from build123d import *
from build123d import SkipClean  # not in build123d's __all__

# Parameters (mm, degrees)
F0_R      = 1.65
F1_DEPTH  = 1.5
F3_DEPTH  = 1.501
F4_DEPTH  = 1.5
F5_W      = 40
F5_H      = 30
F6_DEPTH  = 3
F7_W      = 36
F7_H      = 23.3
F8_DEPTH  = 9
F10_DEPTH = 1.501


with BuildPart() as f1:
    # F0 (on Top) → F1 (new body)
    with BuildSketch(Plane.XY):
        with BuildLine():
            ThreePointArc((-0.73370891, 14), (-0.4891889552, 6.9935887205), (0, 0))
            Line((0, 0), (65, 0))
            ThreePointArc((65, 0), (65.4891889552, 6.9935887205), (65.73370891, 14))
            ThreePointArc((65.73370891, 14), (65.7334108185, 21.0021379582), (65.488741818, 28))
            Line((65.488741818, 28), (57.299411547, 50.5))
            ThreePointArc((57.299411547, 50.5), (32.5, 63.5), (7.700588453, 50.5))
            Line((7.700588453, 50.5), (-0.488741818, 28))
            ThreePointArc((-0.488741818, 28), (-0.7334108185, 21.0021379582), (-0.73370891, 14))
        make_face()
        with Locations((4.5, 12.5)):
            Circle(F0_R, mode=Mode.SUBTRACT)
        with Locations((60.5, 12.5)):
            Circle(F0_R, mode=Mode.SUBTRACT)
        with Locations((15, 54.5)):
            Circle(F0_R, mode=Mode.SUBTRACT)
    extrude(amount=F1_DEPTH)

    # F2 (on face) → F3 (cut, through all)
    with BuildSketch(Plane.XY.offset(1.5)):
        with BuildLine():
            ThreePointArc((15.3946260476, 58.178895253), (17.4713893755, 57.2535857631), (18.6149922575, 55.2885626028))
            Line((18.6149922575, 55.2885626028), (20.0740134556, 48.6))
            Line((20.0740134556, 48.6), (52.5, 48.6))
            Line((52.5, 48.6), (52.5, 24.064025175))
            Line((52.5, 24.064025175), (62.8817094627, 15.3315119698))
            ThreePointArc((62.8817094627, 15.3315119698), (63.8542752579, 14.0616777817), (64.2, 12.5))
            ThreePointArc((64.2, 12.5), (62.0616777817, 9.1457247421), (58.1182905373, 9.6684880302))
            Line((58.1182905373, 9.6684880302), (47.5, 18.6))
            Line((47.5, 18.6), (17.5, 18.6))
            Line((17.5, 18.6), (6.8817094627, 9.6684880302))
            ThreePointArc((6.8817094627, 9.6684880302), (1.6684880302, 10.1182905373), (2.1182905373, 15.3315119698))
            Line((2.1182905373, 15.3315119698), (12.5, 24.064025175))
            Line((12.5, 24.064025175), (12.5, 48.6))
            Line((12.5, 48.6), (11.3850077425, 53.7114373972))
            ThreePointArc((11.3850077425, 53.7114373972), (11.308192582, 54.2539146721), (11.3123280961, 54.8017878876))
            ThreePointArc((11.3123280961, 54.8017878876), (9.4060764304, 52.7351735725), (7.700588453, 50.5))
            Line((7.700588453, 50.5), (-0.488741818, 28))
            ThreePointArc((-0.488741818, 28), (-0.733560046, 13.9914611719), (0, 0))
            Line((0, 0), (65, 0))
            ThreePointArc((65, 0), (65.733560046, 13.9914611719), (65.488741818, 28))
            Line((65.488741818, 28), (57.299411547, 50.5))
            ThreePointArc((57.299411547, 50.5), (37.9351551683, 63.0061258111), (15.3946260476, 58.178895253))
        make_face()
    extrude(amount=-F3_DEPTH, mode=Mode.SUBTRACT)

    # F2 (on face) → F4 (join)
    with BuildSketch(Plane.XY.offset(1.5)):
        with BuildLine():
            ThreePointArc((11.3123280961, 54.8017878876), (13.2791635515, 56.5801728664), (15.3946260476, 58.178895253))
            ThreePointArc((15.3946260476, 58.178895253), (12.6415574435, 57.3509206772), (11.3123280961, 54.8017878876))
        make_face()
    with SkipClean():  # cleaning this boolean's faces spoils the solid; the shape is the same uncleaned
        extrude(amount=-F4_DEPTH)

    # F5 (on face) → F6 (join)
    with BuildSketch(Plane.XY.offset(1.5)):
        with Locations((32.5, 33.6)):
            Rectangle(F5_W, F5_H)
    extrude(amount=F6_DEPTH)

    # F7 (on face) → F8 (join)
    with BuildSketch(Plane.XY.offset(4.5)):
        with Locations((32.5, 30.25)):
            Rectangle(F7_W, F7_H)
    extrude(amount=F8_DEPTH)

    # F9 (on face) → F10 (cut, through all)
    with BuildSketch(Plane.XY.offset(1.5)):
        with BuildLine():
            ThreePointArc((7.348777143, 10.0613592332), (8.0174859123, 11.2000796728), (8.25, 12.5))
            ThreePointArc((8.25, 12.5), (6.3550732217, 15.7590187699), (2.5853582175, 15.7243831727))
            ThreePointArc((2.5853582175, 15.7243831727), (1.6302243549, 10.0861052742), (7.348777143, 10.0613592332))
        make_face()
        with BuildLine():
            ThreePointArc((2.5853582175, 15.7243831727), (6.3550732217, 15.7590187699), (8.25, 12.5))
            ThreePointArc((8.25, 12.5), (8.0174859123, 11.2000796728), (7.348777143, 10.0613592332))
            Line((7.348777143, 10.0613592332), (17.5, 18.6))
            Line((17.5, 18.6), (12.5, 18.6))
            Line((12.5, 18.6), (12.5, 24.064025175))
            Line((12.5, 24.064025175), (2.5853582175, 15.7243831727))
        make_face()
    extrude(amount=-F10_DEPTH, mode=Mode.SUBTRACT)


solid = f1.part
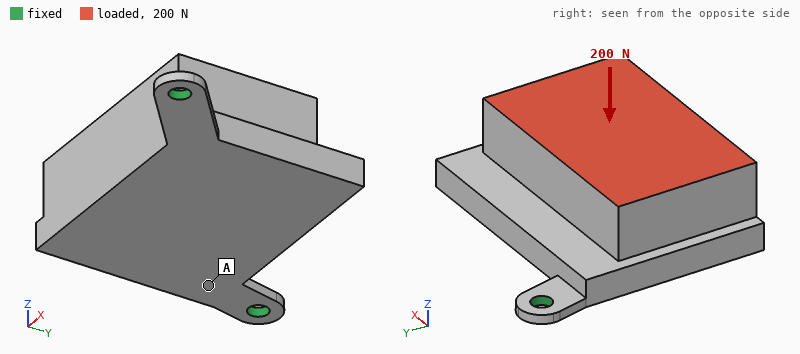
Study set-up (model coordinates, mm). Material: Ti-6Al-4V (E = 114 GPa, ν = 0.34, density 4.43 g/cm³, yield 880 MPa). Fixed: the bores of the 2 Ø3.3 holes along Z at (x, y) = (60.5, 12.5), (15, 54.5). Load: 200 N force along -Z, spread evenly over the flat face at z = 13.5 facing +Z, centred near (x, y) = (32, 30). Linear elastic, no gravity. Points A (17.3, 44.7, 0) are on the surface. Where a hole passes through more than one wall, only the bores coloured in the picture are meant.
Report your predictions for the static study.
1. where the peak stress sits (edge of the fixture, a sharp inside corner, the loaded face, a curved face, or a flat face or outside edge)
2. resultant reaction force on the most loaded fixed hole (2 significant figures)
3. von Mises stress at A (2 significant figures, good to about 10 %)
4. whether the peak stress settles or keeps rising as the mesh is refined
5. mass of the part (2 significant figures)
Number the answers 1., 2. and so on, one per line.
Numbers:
1. edge of the fixture
2. 120 N
3. 22 MPa
4. keeps rising
5. 58 g
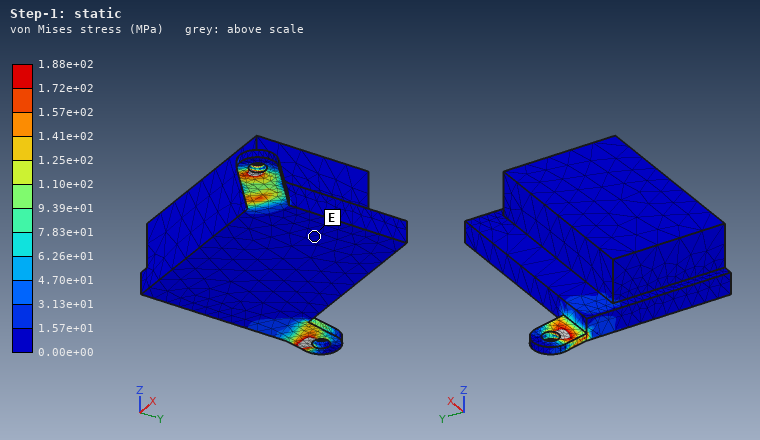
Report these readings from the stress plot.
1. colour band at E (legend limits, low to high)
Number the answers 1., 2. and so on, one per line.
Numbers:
1. 0.00e+00 to 1.57e+01 MPa
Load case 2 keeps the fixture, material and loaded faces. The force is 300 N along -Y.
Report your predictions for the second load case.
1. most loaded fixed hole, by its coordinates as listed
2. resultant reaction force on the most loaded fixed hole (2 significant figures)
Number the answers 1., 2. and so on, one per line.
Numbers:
1. (15, 54.5)
2. 220 N
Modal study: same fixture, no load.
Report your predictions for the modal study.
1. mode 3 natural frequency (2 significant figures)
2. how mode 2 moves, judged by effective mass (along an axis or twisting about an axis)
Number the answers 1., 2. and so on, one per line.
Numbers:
1. 4300 Hz
2. along Z
